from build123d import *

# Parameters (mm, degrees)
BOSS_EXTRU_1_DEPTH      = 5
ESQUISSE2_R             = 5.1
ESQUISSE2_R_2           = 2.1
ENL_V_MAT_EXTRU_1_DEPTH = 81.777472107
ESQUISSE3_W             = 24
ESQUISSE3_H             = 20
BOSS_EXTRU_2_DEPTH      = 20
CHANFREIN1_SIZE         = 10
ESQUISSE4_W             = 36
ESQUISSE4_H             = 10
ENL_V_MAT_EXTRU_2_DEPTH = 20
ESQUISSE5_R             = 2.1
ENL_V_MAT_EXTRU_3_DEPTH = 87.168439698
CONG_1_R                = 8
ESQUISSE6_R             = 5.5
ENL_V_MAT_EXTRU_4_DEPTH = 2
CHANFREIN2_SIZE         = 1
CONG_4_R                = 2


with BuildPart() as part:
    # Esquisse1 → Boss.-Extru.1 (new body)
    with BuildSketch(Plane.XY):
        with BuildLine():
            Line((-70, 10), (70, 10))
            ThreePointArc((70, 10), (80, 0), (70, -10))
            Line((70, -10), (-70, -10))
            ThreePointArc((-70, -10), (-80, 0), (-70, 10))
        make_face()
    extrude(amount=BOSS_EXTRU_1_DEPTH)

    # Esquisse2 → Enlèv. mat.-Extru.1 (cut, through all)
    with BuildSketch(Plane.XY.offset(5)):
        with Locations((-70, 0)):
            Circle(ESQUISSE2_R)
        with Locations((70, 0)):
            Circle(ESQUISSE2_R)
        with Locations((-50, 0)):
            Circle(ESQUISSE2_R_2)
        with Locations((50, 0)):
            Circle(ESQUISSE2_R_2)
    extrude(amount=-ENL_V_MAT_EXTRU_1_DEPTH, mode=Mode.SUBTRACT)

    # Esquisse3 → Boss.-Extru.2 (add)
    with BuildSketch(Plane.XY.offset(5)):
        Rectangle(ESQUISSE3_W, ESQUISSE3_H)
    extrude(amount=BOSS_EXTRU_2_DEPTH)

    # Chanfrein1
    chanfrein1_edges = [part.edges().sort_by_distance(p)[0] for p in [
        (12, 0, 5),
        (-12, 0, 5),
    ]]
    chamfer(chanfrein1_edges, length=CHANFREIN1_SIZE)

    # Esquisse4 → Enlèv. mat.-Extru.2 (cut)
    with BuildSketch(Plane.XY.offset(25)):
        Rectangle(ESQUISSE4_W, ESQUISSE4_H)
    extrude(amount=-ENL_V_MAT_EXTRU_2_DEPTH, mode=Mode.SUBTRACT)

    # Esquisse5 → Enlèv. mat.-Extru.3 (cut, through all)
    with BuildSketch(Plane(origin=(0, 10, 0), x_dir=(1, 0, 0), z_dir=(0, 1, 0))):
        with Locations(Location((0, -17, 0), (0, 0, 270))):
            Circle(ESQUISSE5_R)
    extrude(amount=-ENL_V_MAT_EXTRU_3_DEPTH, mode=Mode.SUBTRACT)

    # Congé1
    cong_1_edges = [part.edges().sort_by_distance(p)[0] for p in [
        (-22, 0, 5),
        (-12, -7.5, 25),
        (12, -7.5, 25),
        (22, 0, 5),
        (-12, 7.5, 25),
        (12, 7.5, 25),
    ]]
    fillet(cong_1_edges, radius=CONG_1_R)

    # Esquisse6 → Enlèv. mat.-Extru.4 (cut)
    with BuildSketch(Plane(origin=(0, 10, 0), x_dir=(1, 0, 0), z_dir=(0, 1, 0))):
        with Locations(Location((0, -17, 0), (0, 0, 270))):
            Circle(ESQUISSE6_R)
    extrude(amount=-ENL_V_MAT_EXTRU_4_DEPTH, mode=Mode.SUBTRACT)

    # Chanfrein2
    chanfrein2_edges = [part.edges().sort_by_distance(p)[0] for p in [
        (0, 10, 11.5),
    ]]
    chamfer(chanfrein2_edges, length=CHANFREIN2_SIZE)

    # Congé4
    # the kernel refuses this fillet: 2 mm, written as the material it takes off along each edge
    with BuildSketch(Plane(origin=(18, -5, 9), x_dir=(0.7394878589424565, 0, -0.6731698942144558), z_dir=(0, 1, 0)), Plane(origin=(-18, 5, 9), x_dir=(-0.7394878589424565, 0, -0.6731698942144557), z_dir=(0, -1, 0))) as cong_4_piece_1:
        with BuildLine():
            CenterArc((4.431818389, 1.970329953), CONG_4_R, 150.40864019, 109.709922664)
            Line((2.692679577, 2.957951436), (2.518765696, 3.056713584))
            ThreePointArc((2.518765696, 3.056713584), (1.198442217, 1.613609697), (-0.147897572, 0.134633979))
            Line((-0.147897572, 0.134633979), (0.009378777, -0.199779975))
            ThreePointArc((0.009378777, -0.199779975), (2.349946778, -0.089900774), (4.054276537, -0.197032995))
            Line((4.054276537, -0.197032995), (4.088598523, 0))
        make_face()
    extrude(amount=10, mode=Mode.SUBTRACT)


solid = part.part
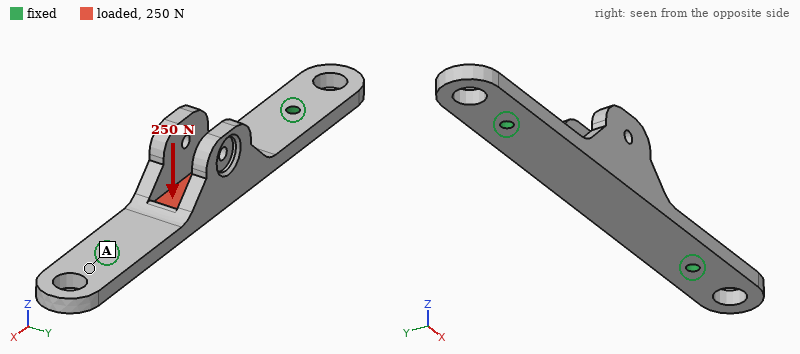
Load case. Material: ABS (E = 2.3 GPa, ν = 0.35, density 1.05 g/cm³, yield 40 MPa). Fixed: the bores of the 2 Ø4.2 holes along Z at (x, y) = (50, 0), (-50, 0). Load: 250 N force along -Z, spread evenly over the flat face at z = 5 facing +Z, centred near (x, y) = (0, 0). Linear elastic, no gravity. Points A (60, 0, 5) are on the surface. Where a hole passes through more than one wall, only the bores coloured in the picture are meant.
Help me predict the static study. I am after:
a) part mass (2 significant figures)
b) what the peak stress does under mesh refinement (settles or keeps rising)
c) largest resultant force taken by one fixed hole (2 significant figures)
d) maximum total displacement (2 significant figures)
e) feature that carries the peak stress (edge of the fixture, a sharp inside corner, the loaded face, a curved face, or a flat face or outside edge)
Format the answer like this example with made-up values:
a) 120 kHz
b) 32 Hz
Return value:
a) 21 g
b) keeps rising
c) 170 N
d) 0.85 mm
e) edge of the fixture
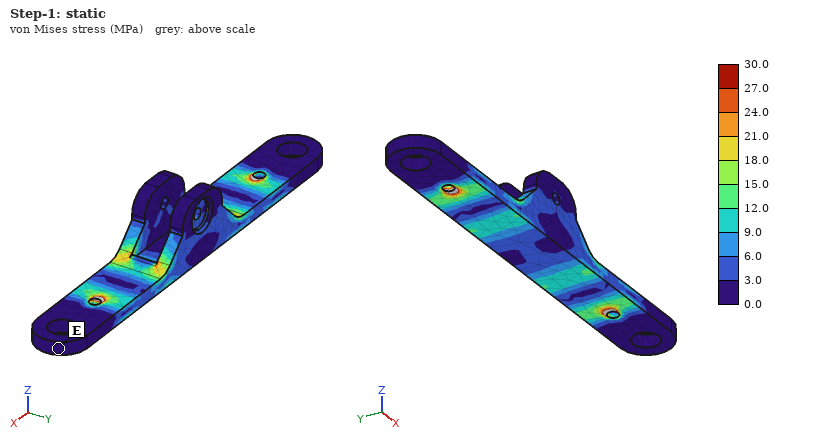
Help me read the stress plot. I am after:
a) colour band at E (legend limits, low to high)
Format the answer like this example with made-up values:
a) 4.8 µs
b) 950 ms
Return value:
a) 0.0 to 3.0 MPa
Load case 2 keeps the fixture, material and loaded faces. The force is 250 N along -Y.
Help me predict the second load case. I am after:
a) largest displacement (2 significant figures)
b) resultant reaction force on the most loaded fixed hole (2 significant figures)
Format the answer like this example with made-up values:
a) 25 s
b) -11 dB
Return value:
a) 0.76 mm
b) 130 N
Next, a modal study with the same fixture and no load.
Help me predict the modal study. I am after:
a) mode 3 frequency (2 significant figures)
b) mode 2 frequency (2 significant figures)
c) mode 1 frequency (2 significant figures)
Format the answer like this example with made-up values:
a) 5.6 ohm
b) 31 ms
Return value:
a) 1600 Hz
b) 810 Hz
c) 790 Hz
